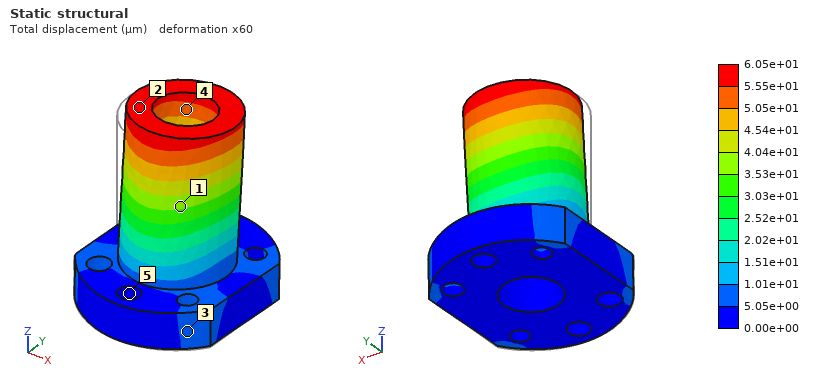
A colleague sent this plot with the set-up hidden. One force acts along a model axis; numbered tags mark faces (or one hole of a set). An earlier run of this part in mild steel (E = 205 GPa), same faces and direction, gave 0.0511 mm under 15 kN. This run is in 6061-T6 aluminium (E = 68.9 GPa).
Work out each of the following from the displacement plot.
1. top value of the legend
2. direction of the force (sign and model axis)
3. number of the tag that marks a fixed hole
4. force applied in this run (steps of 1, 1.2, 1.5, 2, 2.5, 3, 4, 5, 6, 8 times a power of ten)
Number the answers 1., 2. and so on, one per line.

1. 6.05e+01 µm
2. +Y
3. 5
4. 6 kN
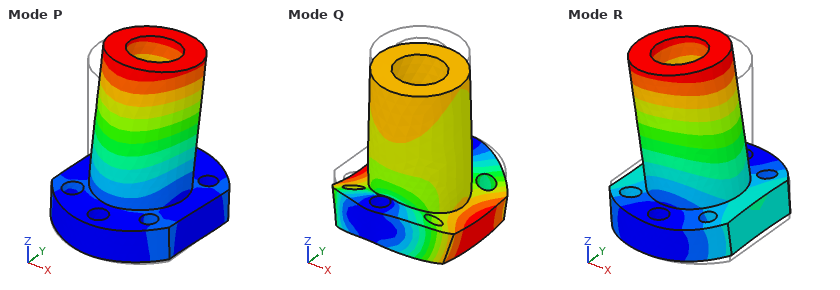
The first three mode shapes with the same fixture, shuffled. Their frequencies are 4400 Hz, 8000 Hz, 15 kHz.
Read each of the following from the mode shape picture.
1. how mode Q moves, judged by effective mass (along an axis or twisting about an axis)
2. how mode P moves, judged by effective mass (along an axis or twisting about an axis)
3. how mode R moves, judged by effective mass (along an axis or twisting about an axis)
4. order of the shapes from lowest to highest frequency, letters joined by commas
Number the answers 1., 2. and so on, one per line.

1. along Z
2. along Y
3. along X
4. R, P, Q
